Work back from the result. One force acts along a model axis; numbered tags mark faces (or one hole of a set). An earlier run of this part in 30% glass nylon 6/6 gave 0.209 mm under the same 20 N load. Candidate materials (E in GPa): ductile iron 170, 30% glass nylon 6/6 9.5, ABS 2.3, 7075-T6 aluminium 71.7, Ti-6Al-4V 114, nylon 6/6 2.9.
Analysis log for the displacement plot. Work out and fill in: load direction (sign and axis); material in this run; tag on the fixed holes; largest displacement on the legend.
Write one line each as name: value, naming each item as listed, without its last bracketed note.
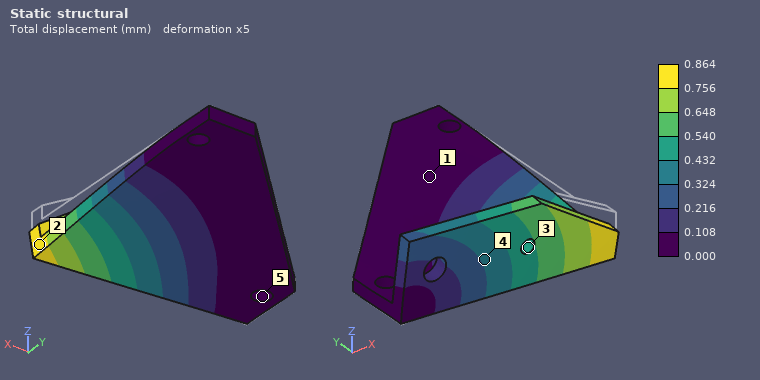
load direction: -Z
material in this run: ABS
tag on the fixed holes: 5
largest displacement on the legend: 0.864 mm
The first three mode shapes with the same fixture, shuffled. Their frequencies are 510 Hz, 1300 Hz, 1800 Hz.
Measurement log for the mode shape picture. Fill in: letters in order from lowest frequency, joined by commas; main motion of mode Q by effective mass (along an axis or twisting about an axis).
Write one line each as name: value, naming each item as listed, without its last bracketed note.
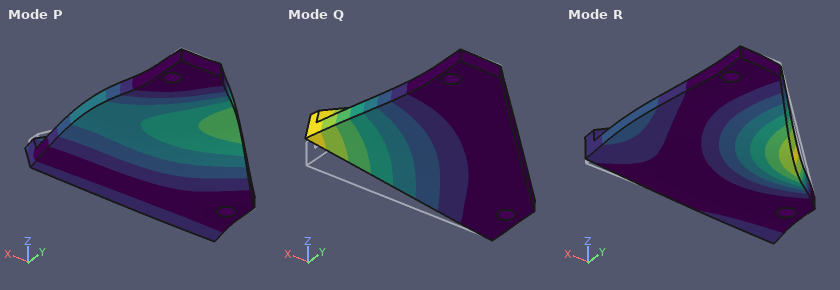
letters in order from lowest frequency, joined by commas: Q, P, R
main motion of mode Q by effective mass: along Z
